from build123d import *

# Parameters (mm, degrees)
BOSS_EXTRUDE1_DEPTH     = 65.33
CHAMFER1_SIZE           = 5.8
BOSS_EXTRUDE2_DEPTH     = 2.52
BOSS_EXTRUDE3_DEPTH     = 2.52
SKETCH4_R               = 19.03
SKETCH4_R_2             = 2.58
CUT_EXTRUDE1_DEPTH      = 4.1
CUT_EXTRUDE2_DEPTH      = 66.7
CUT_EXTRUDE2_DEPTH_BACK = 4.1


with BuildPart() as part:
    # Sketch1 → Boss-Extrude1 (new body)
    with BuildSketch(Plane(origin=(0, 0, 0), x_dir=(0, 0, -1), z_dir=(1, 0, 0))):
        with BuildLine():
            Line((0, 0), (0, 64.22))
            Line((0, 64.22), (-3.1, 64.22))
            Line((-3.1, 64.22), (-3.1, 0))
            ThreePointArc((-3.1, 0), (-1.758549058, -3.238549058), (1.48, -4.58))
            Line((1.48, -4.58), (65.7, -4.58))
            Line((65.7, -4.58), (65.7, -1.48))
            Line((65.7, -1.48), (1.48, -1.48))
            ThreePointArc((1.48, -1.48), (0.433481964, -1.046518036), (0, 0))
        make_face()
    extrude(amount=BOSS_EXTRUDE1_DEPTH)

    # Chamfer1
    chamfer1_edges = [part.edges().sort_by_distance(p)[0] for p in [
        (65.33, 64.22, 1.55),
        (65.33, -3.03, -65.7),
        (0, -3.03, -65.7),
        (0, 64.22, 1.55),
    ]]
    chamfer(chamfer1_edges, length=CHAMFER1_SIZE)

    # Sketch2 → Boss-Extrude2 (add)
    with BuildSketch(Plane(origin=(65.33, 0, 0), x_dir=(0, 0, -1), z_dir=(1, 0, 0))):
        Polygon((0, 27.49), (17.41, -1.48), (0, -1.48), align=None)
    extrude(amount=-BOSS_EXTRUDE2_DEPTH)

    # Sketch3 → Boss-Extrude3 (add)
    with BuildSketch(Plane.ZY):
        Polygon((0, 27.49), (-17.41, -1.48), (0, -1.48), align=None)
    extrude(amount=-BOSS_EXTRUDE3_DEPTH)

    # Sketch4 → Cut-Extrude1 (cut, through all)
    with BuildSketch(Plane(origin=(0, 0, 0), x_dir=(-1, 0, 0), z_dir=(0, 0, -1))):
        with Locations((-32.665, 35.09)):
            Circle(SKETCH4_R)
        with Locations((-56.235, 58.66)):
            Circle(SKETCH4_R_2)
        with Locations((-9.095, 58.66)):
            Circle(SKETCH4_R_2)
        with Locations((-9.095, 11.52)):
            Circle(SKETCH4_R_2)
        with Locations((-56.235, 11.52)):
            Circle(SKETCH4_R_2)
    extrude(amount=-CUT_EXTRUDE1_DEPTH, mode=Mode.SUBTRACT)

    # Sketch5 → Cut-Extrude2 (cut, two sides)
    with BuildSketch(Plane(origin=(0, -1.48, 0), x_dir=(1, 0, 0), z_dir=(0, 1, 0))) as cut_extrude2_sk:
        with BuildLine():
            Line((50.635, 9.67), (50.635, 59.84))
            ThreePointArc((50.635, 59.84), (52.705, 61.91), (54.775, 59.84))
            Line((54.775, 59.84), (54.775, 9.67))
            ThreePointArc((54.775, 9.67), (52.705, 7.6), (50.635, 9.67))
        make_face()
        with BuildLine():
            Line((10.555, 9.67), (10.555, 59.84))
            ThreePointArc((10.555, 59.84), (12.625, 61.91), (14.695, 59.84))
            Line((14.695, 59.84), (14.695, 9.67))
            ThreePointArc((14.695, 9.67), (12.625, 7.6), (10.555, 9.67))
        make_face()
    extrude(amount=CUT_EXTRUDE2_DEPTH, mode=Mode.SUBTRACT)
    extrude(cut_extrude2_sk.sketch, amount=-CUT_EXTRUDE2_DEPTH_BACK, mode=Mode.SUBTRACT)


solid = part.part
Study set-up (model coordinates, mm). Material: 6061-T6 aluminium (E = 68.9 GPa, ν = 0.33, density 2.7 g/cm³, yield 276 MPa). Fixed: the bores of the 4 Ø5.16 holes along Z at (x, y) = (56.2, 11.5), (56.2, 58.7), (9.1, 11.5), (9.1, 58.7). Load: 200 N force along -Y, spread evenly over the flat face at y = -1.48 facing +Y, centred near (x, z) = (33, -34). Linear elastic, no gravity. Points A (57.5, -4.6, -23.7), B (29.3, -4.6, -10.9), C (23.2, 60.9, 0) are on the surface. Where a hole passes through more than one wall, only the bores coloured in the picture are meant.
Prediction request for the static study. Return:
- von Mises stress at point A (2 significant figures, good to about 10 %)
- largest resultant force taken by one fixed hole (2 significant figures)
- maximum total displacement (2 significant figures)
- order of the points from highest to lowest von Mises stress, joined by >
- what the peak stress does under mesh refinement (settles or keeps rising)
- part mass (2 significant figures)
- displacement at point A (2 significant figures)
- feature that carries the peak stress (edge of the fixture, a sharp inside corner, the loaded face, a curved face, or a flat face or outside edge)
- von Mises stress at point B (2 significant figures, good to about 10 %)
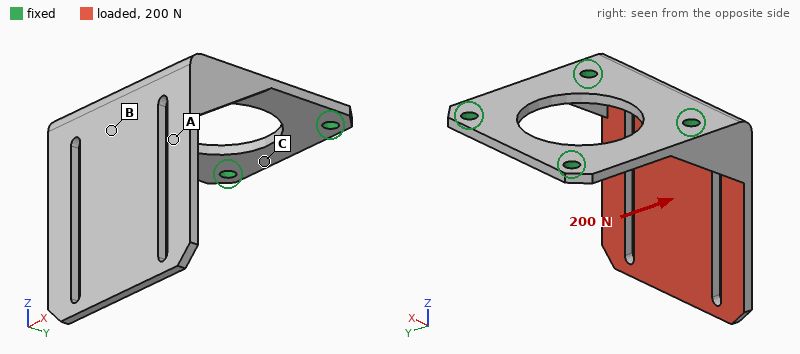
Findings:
51 MPa
110 N
0.71 mm
A > B > C
keeps rising
62 g
0.12 mm
edge of the fixture
27 MPa
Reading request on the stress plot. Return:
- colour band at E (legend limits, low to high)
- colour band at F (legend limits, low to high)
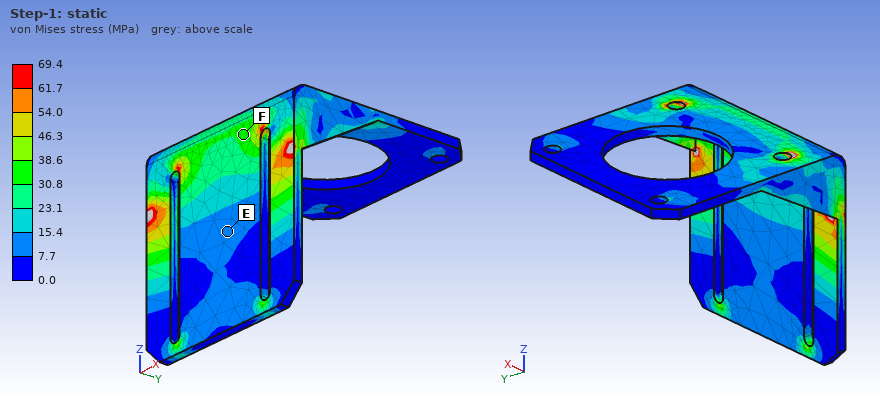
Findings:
7.7 to 15.4 MPa
30.8 to 38.6 MPa
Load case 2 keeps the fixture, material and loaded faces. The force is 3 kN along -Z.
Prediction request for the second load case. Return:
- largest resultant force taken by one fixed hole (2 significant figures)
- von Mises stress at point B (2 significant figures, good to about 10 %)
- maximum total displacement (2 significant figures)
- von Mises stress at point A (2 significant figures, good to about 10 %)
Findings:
1.6 kN
33 MPa
0.30 mm
34 MPa
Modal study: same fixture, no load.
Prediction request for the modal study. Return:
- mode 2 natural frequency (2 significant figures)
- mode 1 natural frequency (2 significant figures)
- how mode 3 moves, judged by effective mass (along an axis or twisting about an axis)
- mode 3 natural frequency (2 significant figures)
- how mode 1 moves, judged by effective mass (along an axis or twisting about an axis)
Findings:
1500 Hz
610 Hz
along X
2400 Hz
along Y
